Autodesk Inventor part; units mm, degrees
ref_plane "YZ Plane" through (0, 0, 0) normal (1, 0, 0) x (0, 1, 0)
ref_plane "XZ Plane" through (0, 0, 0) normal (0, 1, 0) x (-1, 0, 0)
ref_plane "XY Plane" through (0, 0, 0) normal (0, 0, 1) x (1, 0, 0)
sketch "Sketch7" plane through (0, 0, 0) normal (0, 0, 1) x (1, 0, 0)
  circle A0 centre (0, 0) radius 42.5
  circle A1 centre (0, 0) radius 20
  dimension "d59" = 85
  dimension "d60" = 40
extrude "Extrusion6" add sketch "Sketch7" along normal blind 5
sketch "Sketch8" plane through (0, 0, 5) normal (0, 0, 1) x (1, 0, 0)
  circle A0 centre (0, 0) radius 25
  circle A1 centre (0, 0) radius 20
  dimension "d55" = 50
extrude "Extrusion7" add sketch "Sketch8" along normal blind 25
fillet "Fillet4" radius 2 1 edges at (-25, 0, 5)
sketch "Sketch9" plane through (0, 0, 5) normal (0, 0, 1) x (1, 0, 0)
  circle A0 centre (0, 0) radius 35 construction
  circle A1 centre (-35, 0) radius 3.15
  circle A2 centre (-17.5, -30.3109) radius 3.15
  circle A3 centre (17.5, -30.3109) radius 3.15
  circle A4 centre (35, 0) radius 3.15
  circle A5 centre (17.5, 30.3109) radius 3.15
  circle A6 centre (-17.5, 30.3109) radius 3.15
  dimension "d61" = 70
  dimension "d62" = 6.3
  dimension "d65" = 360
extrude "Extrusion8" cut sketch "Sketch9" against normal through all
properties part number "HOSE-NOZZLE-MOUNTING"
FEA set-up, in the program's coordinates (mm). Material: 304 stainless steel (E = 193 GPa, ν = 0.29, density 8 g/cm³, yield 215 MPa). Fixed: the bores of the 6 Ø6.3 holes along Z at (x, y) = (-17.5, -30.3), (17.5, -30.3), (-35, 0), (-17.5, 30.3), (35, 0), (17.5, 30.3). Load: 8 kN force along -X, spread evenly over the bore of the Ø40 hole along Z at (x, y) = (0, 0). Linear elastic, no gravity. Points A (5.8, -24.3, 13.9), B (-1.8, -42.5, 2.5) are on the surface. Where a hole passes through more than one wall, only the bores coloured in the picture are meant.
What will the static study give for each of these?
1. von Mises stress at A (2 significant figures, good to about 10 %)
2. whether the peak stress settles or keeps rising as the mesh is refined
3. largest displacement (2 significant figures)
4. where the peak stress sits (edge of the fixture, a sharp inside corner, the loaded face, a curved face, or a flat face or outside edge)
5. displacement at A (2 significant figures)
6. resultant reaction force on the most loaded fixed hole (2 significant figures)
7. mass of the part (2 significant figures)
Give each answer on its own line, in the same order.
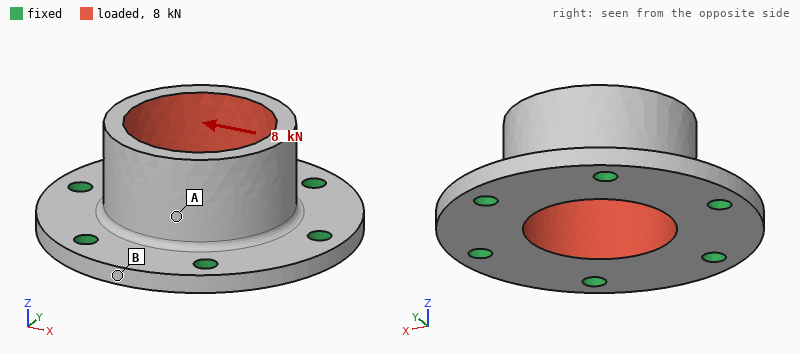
13 MPa
keeps rising
10 µm
edge of the fixture
4.2 µm
2.0 kN
310 g
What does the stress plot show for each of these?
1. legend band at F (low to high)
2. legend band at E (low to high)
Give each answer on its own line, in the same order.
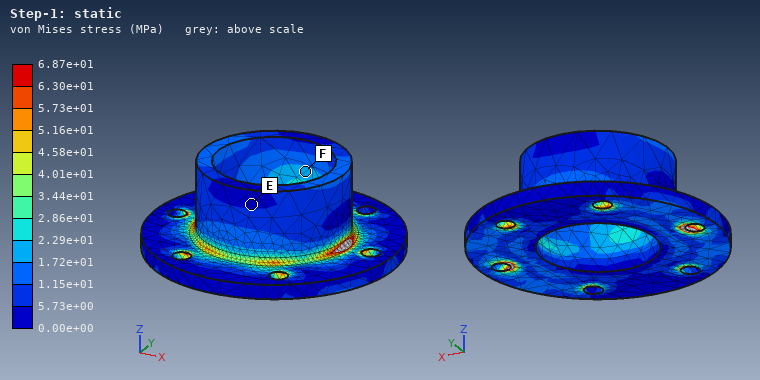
1.72e+01 to 2.29e+01 MPa
0.00e+00 to 5.73e+00 MPa
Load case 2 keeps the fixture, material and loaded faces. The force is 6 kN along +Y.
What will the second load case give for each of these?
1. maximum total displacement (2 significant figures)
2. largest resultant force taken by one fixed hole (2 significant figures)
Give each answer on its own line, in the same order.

7.7 µm
1.3 kN
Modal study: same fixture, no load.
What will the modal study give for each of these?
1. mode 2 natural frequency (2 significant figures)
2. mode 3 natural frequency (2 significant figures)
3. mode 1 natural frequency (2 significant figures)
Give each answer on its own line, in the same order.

11 kHz
11 kHz
11 kHz
